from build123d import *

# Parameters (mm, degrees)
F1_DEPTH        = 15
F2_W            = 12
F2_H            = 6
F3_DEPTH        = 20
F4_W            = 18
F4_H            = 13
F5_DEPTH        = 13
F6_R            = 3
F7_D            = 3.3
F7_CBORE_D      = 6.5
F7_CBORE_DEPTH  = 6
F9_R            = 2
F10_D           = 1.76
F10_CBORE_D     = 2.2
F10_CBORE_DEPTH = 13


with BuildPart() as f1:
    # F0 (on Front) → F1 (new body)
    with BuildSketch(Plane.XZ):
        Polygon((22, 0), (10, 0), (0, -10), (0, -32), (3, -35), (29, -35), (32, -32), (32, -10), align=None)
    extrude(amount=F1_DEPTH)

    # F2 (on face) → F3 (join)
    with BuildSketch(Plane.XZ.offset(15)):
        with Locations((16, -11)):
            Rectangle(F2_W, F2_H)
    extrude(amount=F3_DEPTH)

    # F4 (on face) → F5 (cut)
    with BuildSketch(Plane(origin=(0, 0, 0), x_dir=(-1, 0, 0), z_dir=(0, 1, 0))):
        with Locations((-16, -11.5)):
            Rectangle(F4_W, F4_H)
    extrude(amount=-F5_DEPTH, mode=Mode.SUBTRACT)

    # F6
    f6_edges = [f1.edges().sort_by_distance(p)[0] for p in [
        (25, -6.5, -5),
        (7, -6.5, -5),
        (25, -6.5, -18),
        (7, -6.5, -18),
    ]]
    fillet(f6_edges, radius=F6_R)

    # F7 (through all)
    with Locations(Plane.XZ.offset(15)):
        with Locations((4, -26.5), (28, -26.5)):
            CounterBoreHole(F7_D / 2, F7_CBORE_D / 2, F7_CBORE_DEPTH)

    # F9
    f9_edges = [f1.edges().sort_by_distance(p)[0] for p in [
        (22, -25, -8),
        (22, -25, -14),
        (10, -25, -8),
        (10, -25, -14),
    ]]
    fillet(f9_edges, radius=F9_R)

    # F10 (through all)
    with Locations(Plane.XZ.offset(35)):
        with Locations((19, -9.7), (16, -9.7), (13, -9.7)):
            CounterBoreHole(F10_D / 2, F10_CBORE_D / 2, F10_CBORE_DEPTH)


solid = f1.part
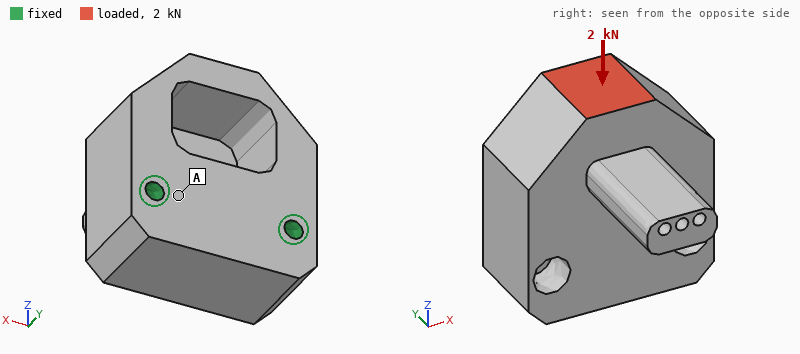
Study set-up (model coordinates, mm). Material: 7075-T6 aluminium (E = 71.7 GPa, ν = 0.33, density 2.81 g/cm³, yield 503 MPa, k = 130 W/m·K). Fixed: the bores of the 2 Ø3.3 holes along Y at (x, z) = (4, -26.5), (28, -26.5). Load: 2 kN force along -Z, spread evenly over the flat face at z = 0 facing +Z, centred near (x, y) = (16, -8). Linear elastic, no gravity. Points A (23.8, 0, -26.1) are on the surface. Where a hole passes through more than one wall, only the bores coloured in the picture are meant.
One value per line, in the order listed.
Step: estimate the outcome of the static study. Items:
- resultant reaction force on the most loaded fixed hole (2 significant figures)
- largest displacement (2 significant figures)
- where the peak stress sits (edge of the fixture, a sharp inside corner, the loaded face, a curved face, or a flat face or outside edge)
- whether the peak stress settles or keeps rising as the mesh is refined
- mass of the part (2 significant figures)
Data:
1.0 kN
22 µm
a sharp inside corner
keeps rising
36 g
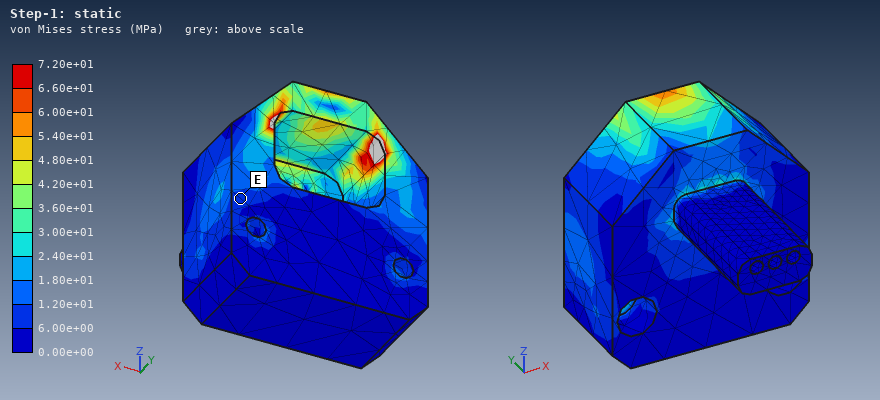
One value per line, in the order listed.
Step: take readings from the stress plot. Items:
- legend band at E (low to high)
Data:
6.00e+00 to 1.20e+01 MPa
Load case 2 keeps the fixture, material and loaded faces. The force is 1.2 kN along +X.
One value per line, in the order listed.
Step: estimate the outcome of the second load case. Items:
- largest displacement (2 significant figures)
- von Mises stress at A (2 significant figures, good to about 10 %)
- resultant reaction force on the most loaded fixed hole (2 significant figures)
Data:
21 µm
11 MPa
1.4 kN
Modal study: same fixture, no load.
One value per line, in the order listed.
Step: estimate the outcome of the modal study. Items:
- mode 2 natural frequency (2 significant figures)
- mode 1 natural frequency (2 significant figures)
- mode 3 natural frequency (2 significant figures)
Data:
11 kHz
6500 Hz
11 kHz
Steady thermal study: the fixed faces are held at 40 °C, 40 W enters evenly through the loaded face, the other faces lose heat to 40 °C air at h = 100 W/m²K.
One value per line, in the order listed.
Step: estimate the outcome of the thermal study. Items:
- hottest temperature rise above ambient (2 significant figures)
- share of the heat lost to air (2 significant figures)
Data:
46 K
18 %
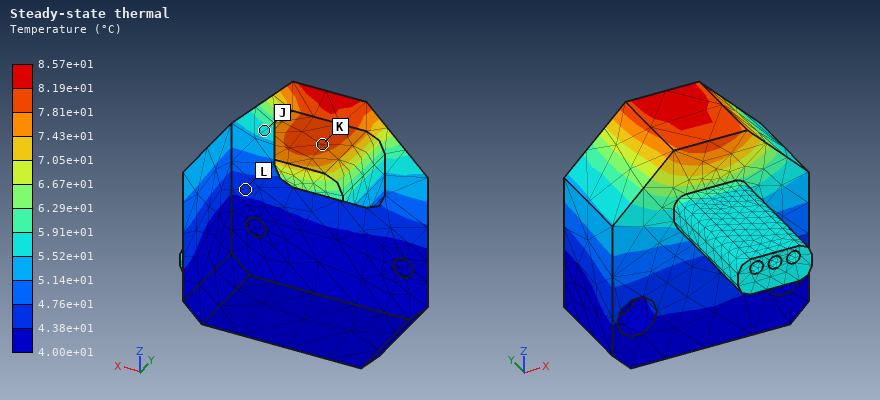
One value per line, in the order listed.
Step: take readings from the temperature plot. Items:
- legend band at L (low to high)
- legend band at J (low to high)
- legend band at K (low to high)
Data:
4.38e+01 to 4.76e+01 °C
5.52e+01 to 5.91e+01 °C
7.81e+01 to 8.19e+01 °C
